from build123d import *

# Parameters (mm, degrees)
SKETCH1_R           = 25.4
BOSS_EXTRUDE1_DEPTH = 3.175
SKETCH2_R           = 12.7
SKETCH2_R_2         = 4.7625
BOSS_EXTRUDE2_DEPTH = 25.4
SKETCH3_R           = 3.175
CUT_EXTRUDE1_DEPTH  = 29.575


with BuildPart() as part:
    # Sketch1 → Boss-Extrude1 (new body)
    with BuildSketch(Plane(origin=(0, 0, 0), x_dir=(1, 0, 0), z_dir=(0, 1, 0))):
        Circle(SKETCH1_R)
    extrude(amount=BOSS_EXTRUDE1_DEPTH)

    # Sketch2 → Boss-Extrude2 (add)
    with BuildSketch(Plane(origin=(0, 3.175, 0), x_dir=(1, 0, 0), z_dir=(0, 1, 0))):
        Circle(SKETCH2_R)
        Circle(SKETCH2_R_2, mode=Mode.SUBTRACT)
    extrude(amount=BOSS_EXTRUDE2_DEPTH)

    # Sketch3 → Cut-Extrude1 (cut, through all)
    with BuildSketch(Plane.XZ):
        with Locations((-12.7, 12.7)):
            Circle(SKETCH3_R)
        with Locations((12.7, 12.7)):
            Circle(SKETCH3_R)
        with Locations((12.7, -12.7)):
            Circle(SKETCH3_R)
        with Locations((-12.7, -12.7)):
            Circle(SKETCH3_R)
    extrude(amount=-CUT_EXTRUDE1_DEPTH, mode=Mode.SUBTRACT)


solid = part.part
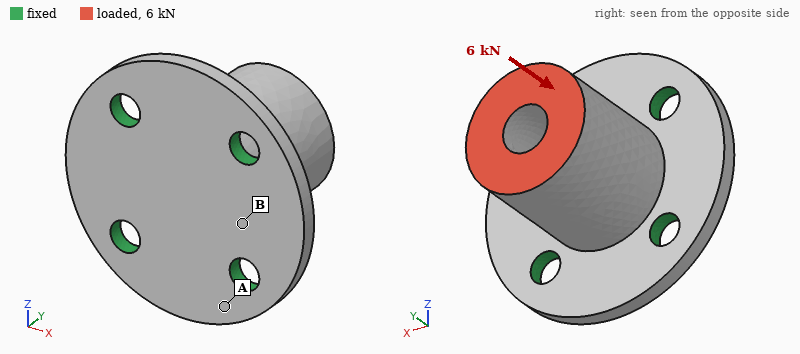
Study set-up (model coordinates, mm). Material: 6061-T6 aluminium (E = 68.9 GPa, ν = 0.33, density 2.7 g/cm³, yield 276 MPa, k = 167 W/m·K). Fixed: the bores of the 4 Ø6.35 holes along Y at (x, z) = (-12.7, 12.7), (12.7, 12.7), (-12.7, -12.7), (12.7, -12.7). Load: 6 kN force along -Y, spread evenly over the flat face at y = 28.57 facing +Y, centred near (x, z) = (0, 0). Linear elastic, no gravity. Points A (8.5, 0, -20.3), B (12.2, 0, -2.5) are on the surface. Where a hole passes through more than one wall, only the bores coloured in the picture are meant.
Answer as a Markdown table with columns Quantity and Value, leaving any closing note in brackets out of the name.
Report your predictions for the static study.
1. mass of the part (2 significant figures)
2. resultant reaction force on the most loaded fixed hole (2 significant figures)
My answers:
| Quantity | Value |
|---|---|
| mass of the part | 46 g |
| resultant reaction force on the most loaded fixed hole | 1.6 kN |
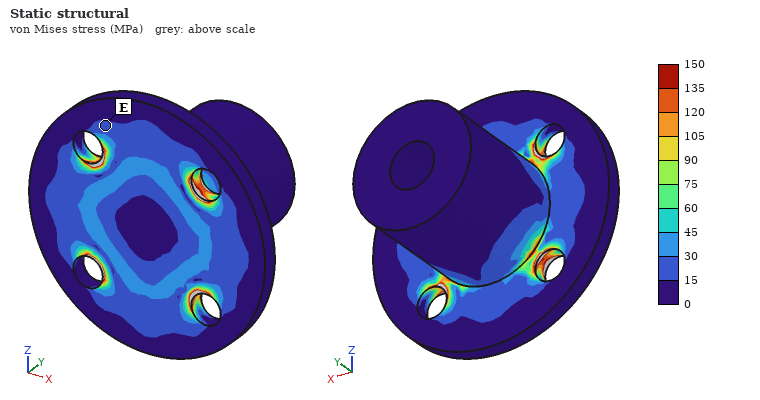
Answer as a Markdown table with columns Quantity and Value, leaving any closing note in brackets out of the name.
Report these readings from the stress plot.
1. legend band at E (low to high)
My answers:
| Quantity | Value |
|---|---|
| legend band at E | 15 to 30 MPa |
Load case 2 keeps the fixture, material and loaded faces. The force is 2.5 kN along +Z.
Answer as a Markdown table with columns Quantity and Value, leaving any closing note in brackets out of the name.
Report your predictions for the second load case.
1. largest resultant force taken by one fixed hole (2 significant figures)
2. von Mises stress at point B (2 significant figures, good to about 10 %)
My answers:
| Quantity | Value |
|---|---|
| largest resultant force taken by one fixed hole | 1.7 kN |
| von Mises stress at point B | 27 MPa |
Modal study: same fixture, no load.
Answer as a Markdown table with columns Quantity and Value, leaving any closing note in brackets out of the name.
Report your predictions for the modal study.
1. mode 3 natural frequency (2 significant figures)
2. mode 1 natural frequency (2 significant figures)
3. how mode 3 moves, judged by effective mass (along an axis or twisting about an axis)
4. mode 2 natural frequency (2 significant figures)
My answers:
| Quantity | Value |
|---|---|
| mode 3 natural frequency | 17 kHz |
| mode 1 natural frequency | 9900 Hz |
| how mode 3 moves, judged by effective mass | along Y |
| mode 2 natural frequency | 9900 Hz |
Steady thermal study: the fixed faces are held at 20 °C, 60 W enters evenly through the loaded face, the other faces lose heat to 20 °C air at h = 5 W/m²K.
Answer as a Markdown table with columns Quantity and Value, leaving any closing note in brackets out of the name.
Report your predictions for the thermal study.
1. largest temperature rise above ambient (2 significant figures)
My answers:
| Quantity | Value |
|---|---|
| largest temperature rise above ambient | 31 K |
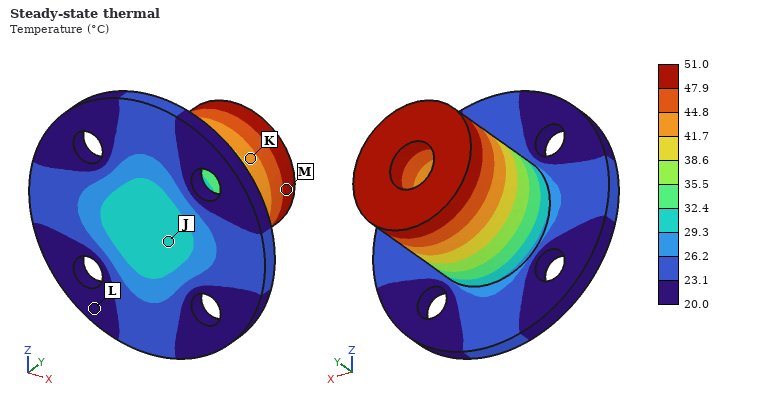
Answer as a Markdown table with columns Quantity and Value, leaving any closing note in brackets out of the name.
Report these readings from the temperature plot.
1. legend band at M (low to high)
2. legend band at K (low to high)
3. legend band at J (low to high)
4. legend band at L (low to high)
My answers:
| Quantity | Value |
|---|---|
| legend band at M | 47.9 to 51.0 °C |
| legend band at K | 41.7 to 44.8 °C |
| legend band at J | 29.3 to 32.4 °C |
| legend band at L | 20.0 to 23.1 °C |
